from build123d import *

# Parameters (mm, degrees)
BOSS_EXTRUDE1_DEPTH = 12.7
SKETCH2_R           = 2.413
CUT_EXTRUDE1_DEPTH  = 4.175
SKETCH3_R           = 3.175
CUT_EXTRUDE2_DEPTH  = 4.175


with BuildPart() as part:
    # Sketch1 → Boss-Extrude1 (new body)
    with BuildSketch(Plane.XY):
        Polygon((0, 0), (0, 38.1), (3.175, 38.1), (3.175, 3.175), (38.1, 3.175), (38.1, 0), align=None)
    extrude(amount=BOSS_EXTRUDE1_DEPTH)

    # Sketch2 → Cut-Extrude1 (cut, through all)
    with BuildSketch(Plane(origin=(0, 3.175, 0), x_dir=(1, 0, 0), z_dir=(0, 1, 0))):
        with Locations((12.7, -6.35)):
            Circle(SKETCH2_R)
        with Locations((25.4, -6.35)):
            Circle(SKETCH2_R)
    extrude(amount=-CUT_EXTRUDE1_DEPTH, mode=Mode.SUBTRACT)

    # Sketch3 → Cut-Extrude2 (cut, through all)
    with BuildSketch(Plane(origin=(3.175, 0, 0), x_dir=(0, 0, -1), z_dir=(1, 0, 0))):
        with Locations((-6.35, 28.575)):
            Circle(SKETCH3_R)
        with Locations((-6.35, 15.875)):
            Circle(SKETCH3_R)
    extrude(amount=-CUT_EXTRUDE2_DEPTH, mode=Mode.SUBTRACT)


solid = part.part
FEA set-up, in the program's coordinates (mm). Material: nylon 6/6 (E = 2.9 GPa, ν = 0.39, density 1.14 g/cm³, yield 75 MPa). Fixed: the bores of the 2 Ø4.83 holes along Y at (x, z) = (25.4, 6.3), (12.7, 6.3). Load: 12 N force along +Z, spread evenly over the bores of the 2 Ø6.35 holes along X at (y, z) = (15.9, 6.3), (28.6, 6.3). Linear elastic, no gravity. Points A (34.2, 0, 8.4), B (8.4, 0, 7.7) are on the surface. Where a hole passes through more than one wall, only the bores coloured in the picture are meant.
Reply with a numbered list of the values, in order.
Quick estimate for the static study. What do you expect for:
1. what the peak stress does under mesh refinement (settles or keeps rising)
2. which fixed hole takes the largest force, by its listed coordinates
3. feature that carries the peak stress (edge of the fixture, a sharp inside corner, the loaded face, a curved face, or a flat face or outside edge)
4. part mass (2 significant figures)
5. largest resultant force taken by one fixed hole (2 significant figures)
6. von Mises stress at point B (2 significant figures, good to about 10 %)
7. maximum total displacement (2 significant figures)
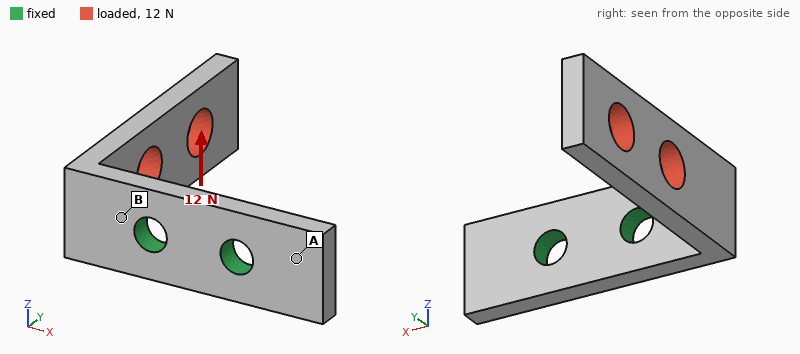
1. keeps rising
2. (12.7, 6.3)
3. edge of the fixture
4. 3.0 g
5. 16 N
6. 7.6 MPa
7. 0.59 mm
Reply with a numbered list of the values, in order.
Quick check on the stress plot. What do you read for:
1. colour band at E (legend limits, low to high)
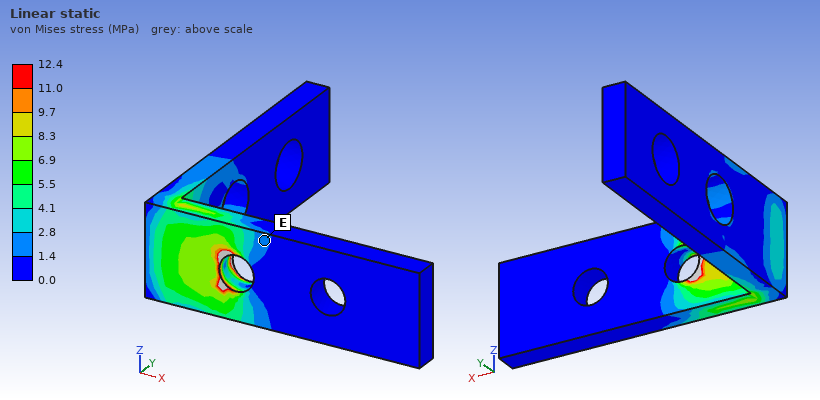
1. 1.4 to 2.8 MPa
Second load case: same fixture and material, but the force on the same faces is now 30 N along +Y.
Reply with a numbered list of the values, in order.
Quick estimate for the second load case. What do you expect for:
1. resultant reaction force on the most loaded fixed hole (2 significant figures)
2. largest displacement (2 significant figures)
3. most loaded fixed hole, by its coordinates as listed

1. 32 N
2. 0.52 mm
3. (12.7, 6.3)
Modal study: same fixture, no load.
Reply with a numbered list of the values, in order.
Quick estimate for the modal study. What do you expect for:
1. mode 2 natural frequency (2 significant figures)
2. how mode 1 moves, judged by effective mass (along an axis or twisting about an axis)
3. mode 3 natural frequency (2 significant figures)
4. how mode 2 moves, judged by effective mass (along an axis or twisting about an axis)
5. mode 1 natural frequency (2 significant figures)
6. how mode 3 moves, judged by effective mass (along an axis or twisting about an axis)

1. 770 Hz
2. along X
3. 2300 Hz
4. along Z
5. 460 Hz
6. along Y
